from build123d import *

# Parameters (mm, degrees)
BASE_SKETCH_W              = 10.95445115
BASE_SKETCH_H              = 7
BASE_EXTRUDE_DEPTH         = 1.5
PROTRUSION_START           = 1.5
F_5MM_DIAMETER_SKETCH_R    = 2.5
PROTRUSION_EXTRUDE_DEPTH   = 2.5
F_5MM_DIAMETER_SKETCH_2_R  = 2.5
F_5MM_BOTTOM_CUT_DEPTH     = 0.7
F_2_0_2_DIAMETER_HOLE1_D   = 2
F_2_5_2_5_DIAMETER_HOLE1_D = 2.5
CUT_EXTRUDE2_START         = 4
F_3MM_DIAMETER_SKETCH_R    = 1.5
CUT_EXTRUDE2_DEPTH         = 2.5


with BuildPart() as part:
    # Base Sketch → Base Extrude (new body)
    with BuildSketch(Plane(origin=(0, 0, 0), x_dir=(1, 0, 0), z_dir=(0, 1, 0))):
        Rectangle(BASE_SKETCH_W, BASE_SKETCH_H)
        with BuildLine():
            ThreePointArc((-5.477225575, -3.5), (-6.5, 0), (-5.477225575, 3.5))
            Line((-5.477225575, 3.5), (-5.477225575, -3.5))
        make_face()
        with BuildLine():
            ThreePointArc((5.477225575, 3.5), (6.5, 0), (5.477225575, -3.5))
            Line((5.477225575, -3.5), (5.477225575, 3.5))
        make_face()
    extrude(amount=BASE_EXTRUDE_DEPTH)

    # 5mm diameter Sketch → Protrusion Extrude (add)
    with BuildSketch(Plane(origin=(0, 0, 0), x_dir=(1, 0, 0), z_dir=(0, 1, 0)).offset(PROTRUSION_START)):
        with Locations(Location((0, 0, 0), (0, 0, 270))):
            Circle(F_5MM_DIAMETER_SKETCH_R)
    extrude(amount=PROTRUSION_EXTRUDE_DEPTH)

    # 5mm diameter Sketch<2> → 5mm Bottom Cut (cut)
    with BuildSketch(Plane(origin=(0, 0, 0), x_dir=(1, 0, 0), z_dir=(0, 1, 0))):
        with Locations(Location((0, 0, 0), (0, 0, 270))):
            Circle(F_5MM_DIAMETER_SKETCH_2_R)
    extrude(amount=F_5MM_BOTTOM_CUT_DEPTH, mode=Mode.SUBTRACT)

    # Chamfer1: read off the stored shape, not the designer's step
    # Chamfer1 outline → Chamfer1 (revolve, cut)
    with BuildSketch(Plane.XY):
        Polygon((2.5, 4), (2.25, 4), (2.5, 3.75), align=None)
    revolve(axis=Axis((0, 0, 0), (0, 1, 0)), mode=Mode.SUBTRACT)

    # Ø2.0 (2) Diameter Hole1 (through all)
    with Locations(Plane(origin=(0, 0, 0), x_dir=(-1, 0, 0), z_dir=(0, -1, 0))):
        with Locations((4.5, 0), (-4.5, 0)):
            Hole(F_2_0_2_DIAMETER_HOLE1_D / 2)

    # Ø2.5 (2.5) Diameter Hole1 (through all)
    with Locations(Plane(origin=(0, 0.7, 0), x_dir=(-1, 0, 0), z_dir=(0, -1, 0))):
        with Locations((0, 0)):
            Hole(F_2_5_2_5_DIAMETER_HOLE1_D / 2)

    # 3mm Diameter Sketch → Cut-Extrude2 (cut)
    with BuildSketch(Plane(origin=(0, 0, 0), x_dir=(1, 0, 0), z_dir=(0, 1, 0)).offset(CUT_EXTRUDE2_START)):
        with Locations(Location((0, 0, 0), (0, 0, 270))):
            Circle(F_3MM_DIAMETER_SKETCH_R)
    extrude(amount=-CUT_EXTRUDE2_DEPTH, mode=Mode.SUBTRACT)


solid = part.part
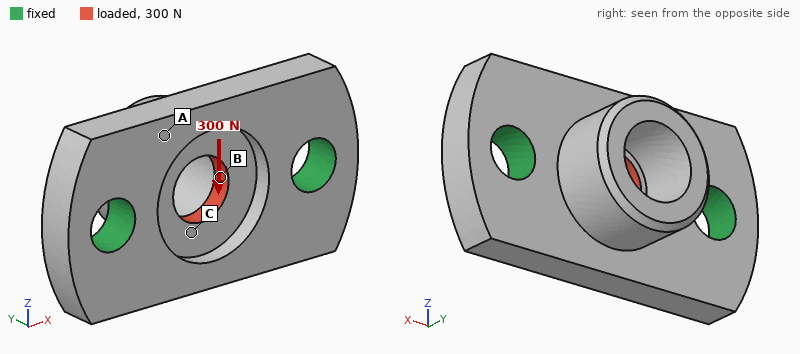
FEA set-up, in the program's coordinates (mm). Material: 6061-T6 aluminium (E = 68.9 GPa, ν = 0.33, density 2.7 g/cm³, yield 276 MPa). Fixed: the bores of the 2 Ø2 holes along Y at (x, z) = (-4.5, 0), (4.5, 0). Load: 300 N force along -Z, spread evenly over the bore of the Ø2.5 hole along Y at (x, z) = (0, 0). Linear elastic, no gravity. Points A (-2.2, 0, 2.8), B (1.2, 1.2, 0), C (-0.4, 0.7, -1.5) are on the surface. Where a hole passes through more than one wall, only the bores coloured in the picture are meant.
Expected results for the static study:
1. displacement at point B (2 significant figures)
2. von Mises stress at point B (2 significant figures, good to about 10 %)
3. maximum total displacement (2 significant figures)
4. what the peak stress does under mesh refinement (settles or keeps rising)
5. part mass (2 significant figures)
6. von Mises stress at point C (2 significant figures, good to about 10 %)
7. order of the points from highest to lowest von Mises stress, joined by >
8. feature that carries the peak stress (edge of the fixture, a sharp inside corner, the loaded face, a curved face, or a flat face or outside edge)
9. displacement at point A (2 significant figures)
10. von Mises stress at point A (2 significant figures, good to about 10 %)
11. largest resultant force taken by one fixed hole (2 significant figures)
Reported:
3.2 µm
84 MPa
3.9 µm
keeps rising
0.36 g
51 MPa
B > C > A
edge of the fixture
1.7 µm
19 MPa
150 N
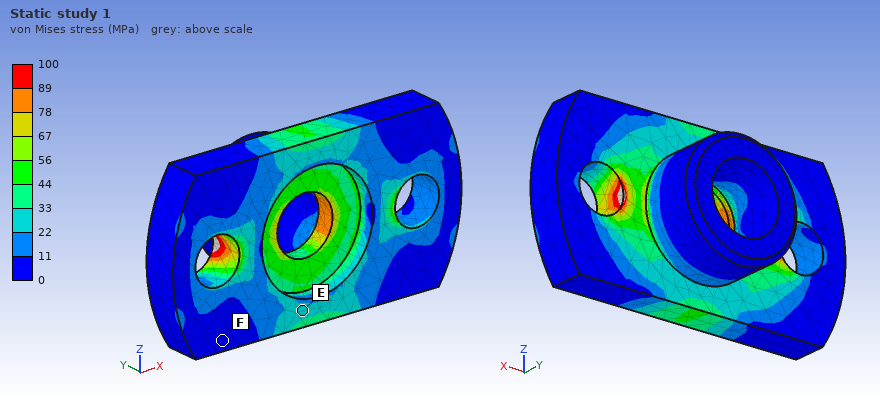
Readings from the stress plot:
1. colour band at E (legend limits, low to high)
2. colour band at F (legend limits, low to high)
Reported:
22 to 33 MPa
0 to 11 MPa
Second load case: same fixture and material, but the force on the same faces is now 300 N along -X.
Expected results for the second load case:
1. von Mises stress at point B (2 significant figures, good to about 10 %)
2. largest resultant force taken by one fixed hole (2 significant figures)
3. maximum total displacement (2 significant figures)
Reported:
44 MPa
150 N
2.1 µm
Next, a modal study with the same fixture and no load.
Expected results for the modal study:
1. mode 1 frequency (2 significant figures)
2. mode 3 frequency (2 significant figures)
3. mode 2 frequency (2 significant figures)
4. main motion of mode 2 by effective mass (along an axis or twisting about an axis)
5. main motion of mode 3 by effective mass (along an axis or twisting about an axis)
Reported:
59 kHz
130 kHz
85 kHz
along Y
along X
